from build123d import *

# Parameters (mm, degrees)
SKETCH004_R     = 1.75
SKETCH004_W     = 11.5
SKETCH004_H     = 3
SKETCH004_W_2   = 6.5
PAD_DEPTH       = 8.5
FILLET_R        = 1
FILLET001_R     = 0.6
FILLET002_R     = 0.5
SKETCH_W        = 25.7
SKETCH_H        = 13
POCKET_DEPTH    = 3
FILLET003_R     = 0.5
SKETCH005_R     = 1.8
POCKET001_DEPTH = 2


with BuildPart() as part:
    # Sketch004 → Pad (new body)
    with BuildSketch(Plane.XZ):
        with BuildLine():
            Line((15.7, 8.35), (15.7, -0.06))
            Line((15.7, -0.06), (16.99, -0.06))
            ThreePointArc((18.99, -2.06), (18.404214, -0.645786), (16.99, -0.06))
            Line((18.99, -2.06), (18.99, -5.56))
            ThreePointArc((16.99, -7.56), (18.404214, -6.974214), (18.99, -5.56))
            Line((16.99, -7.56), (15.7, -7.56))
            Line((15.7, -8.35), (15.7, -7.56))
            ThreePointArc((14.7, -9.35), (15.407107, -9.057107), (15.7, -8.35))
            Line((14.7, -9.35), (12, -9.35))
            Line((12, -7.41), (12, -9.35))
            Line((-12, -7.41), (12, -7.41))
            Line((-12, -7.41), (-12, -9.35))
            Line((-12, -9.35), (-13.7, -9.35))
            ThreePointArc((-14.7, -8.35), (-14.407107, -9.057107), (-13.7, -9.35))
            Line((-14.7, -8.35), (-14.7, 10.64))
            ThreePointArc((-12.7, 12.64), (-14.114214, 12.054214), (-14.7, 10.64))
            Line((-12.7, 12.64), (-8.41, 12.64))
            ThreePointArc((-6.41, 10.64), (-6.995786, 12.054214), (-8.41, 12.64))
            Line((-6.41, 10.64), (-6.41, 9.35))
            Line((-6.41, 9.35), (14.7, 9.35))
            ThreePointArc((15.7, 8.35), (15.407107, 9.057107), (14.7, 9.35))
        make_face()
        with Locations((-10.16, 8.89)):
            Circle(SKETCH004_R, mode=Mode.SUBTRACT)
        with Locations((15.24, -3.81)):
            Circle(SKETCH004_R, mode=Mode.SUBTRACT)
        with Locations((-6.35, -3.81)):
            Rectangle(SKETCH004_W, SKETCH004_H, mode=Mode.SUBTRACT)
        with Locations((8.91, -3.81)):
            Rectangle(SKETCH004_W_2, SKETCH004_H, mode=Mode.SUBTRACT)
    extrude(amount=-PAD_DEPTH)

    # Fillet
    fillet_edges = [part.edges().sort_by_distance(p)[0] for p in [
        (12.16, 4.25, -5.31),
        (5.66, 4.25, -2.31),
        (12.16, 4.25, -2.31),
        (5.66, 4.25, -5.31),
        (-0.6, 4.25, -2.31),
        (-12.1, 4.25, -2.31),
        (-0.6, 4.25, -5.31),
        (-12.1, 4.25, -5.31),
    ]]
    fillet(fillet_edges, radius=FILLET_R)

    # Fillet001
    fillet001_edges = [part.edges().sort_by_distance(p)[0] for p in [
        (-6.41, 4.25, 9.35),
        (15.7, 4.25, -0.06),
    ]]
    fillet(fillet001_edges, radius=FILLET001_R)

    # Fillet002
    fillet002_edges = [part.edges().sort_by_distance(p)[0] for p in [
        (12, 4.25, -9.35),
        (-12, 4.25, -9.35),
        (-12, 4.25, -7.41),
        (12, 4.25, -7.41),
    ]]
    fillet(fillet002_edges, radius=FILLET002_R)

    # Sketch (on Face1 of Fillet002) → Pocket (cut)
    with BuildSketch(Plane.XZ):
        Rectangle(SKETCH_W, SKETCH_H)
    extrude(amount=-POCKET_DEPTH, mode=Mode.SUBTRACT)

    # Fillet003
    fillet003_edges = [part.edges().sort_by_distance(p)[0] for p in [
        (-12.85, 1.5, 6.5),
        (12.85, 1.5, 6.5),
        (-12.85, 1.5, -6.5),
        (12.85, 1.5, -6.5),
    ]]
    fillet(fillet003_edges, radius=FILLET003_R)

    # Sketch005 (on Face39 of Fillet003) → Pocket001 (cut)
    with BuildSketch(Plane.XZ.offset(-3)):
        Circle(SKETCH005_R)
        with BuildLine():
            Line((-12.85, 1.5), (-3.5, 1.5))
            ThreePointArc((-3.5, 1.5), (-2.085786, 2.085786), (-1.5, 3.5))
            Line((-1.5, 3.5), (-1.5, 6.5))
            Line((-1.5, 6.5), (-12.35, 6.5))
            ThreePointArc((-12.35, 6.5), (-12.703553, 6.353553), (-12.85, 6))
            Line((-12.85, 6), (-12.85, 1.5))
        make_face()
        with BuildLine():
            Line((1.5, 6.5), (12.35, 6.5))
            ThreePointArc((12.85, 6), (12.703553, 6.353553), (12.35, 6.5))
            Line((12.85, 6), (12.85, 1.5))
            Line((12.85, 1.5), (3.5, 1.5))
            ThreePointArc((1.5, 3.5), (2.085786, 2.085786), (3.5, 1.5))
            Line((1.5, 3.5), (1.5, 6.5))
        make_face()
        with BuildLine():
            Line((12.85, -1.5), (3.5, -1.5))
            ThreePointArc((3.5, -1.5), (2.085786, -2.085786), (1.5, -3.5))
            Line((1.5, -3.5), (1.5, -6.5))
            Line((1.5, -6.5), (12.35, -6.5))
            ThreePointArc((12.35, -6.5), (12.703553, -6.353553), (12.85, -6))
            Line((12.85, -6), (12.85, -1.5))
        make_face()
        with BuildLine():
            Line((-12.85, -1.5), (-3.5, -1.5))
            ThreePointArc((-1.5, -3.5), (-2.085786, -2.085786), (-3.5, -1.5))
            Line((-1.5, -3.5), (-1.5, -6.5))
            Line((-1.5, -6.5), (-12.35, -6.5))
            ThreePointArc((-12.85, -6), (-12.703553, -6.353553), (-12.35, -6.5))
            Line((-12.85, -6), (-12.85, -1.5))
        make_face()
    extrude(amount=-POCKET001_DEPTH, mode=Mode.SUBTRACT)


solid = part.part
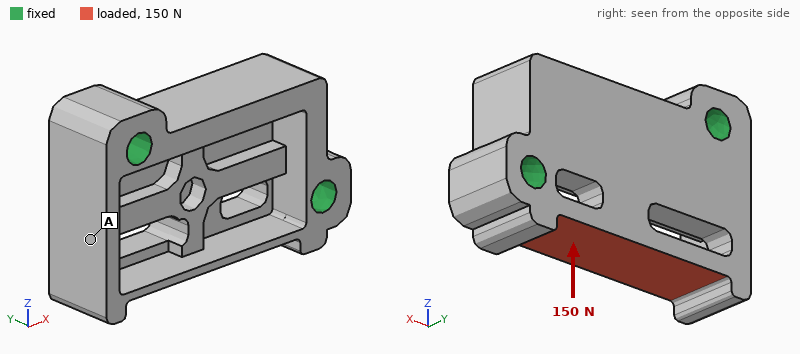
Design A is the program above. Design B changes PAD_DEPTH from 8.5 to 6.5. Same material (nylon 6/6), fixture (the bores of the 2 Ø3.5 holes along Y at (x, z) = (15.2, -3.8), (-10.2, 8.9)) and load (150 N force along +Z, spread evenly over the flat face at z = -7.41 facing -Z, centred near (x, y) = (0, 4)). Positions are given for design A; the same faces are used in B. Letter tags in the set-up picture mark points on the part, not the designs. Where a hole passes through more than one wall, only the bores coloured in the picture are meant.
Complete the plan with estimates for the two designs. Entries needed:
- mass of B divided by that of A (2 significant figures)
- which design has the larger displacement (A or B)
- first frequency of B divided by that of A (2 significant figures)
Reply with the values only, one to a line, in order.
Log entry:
0.67
B
0.80
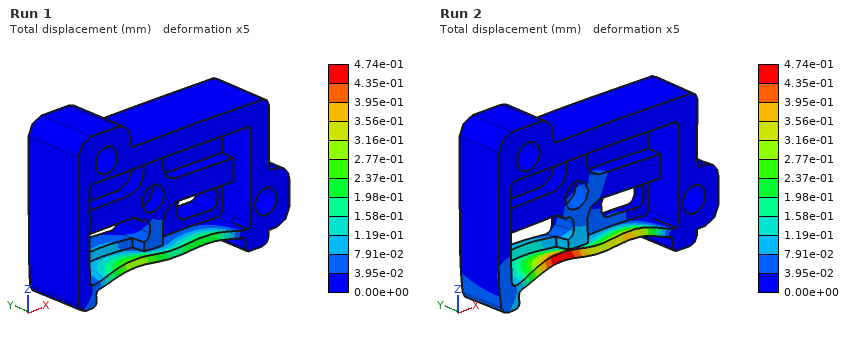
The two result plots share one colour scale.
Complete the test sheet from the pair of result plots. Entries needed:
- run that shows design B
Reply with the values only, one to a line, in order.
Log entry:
Run 2
